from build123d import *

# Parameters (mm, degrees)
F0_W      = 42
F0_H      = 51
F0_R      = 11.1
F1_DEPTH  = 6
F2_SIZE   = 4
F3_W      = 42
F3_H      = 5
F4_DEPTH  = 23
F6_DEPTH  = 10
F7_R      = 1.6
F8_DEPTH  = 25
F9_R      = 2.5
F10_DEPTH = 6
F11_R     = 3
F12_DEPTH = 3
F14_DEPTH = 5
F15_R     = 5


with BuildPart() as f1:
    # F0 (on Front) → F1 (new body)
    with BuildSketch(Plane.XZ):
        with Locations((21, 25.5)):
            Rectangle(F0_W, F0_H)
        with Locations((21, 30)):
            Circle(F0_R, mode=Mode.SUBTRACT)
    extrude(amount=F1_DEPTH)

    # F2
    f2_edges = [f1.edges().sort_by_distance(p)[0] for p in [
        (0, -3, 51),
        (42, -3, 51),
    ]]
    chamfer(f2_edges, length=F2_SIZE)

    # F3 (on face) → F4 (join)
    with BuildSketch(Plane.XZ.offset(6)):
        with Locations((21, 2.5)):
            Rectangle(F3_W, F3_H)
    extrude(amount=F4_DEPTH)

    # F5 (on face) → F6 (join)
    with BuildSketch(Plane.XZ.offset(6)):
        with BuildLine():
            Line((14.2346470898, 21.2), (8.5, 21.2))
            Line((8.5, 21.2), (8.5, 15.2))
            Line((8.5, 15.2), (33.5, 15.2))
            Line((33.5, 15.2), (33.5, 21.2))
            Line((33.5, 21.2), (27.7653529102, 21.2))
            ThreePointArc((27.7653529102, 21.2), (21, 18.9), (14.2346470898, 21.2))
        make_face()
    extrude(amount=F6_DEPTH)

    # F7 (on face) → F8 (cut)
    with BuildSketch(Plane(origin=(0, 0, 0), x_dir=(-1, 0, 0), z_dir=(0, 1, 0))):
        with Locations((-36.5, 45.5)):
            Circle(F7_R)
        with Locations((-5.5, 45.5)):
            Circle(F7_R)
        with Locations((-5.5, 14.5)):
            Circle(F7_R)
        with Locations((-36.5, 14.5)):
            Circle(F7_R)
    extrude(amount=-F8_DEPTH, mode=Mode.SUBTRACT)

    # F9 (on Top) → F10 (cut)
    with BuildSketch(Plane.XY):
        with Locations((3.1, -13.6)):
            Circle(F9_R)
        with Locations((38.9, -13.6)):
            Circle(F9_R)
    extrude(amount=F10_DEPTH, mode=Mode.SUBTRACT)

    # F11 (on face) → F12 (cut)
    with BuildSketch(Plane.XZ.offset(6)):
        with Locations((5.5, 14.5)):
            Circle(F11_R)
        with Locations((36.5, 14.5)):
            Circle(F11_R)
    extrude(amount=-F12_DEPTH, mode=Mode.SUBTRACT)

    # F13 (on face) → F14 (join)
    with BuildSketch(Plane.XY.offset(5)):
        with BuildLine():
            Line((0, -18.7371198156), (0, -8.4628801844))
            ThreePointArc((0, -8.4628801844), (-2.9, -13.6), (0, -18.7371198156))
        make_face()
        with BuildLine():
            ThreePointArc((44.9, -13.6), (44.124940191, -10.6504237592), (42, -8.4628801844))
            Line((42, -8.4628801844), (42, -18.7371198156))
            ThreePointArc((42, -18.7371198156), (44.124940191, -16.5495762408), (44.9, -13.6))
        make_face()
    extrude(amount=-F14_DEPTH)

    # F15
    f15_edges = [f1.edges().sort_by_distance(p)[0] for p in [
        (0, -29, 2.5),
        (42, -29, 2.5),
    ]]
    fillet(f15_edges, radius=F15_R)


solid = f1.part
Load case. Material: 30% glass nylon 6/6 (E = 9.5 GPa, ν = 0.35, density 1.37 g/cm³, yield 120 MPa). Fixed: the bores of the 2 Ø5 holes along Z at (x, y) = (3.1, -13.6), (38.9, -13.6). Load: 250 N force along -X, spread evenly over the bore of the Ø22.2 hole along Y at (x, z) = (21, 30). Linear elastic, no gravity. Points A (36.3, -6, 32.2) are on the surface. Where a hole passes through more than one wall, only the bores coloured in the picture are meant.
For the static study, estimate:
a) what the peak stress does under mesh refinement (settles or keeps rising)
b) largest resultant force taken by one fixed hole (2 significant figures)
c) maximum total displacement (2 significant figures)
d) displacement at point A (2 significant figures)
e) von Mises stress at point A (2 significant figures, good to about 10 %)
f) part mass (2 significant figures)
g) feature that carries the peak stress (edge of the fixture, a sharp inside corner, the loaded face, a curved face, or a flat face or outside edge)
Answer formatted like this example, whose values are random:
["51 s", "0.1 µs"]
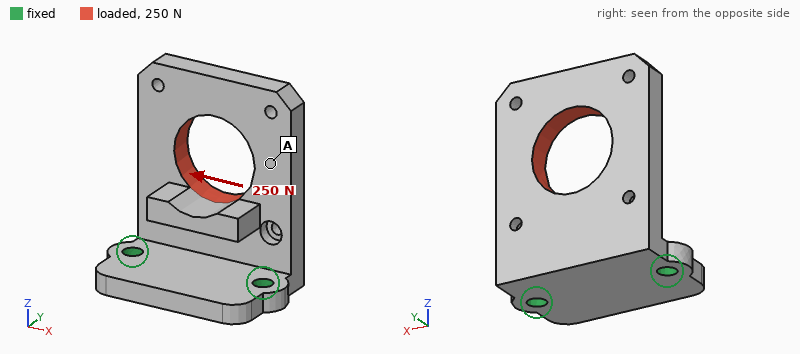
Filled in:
["keeps rising", "240 N", "0.13 mm", "0.086 mm", "2.5 MPa", "22 g", "edge of the fixture"]
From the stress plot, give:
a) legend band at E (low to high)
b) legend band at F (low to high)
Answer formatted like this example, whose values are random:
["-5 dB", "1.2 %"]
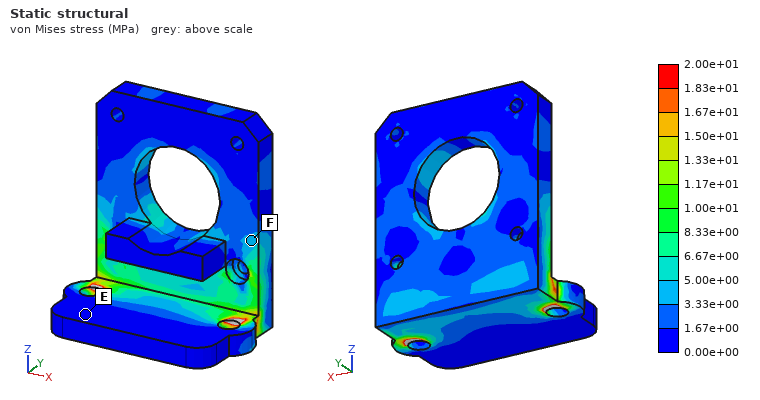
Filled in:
["0.00e+00 to 1.67e+00 MPa", "3.33e+00 to 5.00e+00 MPa"]
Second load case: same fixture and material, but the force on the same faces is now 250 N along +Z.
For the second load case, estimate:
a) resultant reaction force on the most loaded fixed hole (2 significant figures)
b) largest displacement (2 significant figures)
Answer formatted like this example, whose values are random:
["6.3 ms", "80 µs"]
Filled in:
["130 N", "0.17 mm"]
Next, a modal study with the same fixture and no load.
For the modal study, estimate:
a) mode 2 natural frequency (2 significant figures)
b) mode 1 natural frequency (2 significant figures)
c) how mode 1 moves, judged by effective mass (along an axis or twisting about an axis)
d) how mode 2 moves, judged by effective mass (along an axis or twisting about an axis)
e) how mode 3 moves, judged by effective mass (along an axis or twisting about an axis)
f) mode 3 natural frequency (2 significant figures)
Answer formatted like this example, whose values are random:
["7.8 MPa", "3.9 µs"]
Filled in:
["2100 Hz", "760 Hz", "along Y", "along X", "along X", "2700 Hz"]
